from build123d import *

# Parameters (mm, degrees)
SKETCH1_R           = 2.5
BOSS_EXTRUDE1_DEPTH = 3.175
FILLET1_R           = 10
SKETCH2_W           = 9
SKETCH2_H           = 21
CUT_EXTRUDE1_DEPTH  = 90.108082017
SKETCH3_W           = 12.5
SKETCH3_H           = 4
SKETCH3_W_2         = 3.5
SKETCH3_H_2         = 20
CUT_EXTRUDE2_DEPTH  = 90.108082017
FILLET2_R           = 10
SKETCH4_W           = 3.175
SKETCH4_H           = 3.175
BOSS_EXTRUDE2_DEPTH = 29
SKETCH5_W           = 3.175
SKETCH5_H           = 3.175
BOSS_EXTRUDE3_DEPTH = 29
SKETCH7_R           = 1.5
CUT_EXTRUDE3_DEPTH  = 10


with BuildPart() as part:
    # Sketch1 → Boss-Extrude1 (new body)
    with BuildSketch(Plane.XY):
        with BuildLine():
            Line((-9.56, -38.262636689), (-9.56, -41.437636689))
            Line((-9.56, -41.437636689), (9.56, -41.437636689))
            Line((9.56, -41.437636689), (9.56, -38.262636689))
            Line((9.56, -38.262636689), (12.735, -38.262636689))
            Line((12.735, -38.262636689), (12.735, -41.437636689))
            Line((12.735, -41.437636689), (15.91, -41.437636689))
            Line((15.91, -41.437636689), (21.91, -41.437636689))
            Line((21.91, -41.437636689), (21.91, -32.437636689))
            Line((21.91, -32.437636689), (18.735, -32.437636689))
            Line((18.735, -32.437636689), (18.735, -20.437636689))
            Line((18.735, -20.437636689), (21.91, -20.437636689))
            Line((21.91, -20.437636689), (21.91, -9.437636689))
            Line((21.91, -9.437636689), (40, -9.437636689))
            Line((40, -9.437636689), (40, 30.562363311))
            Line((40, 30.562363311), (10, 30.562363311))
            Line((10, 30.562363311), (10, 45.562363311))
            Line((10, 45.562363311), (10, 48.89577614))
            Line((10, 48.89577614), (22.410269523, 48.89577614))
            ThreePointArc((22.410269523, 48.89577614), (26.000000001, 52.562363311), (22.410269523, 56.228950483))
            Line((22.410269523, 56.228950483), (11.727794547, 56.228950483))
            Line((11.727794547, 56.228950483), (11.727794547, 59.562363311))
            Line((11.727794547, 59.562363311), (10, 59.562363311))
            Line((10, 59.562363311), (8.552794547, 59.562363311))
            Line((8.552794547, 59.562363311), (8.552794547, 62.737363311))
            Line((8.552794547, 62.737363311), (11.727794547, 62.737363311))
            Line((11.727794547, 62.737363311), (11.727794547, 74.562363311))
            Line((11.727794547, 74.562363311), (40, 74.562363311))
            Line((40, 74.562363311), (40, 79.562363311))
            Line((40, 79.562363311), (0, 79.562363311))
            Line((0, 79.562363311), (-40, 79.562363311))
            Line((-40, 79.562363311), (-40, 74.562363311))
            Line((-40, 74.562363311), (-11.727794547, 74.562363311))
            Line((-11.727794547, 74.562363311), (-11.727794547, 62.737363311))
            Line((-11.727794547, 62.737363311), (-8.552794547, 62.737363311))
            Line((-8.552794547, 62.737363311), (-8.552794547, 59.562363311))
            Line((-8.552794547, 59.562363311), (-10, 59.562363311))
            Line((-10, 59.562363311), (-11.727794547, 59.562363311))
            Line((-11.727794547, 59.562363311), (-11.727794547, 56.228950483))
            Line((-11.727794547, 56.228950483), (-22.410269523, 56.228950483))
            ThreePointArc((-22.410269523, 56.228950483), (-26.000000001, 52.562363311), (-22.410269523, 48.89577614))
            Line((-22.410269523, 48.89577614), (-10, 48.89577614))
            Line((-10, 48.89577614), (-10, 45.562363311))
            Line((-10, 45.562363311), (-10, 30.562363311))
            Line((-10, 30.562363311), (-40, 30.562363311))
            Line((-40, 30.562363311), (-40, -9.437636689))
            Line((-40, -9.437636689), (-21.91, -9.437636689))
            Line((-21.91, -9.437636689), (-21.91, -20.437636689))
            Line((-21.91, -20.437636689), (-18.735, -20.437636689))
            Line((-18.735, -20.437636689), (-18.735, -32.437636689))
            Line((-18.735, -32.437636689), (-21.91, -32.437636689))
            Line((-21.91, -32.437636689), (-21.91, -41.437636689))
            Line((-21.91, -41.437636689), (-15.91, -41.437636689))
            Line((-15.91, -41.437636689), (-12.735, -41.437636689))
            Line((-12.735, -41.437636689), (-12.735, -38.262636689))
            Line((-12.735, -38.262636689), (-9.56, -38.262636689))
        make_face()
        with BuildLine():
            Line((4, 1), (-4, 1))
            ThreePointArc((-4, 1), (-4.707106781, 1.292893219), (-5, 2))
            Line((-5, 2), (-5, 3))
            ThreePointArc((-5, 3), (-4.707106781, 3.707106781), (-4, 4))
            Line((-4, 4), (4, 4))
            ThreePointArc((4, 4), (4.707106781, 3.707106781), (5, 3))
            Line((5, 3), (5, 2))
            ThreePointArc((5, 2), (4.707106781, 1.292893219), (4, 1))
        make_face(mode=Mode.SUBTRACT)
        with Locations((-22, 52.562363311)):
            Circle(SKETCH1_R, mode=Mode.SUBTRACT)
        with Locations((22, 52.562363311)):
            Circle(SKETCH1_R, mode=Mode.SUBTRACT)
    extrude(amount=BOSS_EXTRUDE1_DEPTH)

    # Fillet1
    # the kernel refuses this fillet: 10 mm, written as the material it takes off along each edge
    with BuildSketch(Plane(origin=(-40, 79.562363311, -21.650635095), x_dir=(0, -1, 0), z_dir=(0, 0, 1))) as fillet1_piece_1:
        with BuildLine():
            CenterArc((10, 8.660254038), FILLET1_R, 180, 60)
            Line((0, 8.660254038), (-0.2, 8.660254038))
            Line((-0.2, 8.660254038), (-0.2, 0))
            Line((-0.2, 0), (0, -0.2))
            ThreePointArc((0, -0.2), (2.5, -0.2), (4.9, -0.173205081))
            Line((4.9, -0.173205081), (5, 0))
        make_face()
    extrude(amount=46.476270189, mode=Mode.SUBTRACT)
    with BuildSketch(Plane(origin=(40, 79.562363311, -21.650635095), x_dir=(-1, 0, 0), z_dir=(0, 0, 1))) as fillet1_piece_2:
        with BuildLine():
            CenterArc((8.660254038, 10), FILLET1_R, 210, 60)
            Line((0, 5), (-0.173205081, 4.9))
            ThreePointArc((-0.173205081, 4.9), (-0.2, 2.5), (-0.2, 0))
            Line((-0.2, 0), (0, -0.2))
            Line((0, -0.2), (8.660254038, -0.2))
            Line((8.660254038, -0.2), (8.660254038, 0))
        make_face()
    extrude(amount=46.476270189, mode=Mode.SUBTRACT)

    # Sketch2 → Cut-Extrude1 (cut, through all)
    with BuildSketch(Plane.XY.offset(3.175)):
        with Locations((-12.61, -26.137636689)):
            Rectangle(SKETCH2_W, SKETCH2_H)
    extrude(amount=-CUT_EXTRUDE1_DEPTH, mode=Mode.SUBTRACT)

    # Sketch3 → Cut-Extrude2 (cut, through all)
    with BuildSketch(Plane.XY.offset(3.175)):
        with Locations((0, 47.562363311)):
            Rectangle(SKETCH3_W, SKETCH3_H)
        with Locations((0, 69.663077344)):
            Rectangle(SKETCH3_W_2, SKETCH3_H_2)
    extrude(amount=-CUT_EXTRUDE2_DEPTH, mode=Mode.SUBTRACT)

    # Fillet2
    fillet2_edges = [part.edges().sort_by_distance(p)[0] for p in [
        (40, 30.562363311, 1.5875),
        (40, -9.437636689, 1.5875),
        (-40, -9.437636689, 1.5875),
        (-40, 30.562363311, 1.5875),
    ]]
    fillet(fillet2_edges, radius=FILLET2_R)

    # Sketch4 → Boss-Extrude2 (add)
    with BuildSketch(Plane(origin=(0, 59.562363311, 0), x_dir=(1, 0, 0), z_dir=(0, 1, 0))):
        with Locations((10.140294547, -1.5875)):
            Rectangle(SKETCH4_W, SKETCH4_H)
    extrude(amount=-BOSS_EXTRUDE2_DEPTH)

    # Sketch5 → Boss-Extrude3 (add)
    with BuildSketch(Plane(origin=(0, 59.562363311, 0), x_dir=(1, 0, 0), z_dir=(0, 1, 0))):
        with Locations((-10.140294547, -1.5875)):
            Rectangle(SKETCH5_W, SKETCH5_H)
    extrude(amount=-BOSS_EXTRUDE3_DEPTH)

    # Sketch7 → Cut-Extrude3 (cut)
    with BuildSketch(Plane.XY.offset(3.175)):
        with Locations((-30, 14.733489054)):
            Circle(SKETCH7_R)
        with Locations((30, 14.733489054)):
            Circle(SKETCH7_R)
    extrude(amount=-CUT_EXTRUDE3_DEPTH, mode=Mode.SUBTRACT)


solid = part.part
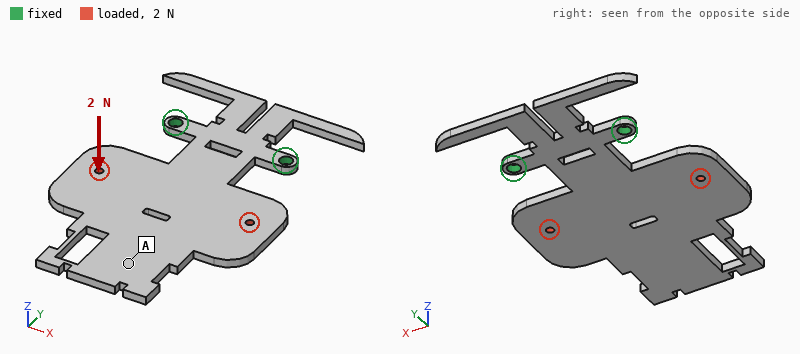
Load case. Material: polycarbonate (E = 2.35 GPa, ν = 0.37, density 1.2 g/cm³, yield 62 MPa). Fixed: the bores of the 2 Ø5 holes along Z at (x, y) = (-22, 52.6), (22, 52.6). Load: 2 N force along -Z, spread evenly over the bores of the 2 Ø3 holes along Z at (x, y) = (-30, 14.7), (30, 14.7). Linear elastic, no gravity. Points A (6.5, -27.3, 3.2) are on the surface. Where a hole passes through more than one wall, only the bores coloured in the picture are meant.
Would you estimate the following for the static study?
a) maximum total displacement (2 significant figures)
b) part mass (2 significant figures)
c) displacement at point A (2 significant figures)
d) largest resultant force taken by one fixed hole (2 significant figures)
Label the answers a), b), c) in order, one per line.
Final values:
a) 1.6 mm
b) 21 g
c) 1.4 mm
d) 1.0 N
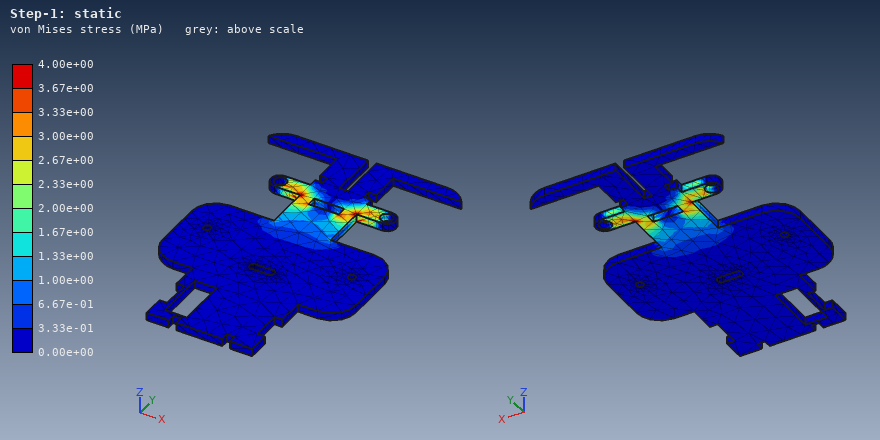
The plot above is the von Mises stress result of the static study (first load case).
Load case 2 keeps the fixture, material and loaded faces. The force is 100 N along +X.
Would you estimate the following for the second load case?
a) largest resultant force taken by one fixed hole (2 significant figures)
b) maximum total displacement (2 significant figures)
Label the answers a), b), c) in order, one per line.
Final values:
a) 120 N
b) 1.5 mm
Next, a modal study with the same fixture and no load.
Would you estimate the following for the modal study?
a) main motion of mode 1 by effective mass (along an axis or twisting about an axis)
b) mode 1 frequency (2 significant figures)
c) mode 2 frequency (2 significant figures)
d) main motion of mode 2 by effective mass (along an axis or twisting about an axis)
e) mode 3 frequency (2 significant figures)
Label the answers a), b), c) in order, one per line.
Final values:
a) along Z
b) 46 Hz
c) 160 Hz
d) twisting about Y
e) 310 Hz
